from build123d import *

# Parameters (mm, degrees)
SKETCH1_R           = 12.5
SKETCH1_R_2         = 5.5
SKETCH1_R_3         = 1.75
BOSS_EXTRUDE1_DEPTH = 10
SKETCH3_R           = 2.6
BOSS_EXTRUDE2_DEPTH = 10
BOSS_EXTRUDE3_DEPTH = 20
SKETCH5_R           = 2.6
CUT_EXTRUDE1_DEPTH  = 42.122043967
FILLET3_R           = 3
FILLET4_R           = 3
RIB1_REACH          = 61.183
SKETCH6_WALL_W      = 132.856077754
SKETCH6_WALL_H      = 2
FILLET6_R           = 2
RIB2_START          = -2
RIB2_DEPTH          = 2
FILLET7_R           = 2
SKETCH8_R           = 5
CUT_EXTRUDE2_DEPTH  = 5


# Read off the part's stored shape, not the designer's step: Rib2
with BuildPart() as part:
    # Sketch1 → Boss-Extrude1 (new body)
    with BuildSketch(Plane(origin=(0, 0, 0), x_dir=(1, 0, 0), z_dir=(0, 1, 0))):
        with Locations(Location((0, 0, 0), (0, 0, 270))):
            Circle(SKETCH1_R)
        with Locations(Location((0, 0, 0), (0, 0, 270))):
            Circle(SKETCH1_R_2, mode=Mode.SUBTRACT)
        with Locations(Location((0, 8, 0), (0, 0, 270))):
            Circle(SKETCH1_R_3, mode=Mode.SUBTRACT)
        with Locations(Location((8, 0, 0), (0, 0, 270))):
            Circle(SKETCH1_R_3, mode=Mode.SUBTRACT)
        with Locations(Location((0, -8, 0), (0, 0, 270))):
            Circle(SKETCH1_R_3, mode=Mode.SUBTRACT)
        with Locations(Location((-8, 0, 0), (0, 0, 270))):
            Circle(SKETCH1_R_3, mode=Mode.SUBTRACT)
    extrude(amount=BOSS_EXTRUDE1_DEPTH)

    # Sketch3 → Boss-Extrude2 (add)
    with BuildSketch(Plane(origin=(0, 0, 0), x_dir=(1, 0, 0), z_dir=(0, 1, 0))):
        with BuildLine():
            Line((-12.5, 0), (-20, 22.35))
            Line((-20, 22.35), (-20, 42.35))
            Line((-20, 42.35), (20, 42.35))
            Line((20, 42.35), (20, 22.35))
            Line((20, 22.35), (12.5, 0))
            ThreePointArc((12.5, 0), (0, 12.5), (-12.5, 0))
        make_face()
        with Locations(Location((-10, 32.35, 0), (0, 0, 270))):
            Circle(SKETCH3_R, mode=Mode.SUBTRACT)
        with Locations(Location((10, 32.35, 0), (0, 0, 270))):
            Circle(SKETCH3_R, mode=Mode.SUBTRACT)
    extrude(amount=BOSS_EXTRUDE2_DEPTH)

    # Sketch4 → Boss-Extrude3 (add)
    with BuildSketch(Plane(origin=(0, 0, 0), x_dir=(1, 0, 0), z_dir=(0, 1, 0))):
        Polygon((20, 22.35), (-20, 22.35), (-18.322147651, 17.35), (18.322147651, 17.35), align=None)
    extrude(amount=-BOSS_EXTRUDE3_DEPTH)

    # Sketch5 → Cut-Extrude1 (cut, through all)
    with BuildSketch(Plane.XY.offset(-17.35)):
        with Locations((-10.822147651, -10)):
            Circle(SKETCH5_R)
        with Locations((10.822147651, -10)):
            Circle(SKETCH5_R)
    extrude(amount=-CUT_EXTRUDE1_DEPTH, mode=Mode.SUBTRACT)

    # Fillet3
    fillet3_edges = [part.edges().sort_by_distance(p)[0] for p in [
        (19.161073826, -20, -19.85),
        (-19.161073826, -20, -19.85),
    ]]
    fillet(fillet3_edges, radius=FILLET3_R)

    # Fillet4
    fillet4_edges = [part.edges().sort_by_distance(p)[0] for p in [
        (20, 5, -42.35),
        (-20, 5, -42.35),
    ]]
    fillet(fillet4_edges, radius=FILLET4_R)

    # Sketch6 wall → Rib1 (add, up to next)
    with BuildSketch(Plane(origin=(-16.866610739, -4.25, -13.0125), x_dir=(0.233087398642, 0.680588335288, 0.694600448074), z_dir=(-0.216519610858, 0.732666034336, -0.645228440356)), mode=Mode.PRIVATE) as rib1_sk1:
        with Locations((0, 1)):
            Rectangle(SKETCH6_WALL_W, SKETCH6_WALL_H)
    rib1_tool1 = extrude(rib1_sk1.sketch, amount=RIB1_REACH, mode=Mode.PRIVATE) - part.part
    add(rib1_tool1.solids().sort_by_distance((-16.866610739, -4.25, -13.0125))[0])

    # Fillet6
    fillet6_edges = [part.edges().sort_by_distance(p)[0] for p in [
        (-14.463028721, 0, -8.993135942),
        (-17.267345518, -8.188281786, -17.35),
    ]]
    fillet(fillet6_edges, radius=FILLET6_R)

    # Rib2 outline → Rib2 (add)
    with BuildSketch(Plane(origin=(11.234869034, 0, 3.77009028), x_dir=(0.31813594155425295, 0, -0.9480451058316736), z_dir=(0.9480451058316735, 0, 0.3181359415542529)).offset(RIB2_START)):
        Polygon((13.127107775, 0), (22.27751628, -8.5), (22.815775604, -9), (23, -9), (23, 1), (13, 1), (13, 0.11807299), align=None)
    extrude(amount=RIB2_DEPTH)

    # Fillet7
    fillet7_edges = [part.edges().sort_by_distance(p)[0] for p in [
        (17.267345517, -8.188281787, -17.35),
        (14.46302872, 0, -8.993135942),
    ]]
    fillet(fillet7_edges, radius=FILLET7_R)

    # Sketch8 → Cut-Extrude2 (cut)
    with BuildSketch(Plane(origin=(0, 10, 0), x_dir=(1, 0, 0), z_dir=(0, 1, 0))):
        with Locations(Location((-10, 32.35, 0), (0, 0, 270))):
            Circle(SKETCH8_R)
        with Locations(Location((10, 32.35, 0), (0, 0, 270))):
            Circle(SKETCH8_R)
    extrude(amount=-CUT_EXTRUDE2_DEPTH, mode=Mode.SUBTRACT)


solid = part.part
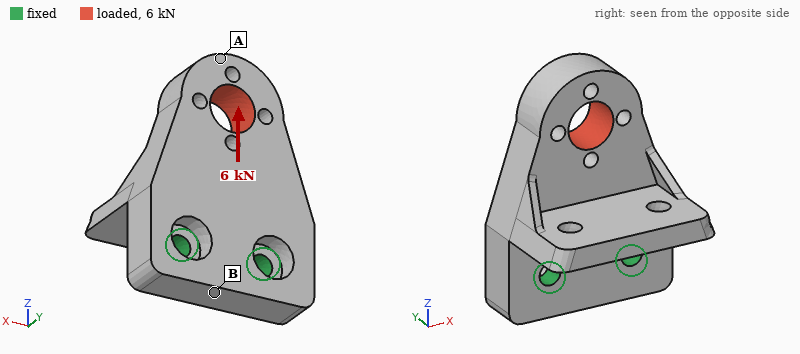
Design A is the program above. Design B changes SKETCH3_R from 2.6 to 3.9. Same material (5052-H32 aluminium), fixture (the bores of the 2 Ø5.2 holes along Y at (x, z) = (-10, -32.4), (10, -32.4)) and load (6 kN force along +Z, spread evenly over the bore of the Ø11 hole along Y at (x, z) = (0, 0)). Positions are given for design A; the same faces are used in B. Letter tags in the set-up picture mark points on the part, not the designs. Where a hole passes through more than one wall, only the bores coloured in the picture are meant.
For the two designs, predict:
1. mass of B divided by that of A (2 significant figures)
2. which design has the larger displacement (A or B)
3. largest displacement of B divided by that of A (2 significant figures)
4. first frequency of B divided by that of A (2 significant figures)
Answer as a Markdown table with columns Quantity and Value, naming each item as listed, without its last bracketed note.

| Quantity | Value |
|---|---|
| mass of B divided by that of A | 0.99 |
| which design has the larger displacement | A |
| largest displacement of B divided by that of A | 0.66 |
| first frequency of B divided by that of A | 1.2 |
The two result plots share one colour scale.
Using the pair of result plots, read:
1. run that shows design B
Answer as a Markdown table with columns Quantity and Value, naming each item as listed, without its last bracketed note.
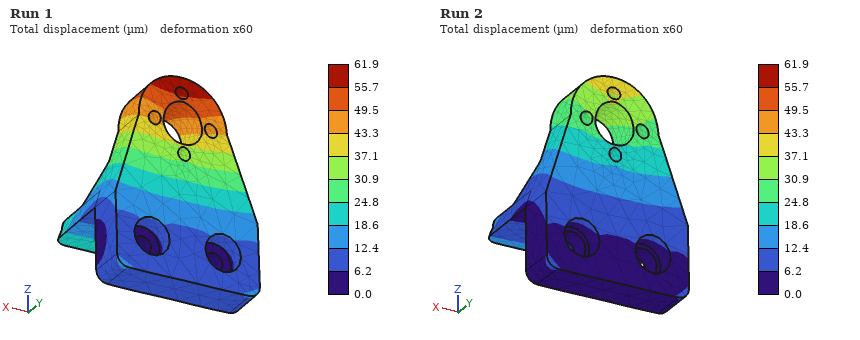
| Quantity | Value |
|---|---|
| run that shows design B | Run 2 |
